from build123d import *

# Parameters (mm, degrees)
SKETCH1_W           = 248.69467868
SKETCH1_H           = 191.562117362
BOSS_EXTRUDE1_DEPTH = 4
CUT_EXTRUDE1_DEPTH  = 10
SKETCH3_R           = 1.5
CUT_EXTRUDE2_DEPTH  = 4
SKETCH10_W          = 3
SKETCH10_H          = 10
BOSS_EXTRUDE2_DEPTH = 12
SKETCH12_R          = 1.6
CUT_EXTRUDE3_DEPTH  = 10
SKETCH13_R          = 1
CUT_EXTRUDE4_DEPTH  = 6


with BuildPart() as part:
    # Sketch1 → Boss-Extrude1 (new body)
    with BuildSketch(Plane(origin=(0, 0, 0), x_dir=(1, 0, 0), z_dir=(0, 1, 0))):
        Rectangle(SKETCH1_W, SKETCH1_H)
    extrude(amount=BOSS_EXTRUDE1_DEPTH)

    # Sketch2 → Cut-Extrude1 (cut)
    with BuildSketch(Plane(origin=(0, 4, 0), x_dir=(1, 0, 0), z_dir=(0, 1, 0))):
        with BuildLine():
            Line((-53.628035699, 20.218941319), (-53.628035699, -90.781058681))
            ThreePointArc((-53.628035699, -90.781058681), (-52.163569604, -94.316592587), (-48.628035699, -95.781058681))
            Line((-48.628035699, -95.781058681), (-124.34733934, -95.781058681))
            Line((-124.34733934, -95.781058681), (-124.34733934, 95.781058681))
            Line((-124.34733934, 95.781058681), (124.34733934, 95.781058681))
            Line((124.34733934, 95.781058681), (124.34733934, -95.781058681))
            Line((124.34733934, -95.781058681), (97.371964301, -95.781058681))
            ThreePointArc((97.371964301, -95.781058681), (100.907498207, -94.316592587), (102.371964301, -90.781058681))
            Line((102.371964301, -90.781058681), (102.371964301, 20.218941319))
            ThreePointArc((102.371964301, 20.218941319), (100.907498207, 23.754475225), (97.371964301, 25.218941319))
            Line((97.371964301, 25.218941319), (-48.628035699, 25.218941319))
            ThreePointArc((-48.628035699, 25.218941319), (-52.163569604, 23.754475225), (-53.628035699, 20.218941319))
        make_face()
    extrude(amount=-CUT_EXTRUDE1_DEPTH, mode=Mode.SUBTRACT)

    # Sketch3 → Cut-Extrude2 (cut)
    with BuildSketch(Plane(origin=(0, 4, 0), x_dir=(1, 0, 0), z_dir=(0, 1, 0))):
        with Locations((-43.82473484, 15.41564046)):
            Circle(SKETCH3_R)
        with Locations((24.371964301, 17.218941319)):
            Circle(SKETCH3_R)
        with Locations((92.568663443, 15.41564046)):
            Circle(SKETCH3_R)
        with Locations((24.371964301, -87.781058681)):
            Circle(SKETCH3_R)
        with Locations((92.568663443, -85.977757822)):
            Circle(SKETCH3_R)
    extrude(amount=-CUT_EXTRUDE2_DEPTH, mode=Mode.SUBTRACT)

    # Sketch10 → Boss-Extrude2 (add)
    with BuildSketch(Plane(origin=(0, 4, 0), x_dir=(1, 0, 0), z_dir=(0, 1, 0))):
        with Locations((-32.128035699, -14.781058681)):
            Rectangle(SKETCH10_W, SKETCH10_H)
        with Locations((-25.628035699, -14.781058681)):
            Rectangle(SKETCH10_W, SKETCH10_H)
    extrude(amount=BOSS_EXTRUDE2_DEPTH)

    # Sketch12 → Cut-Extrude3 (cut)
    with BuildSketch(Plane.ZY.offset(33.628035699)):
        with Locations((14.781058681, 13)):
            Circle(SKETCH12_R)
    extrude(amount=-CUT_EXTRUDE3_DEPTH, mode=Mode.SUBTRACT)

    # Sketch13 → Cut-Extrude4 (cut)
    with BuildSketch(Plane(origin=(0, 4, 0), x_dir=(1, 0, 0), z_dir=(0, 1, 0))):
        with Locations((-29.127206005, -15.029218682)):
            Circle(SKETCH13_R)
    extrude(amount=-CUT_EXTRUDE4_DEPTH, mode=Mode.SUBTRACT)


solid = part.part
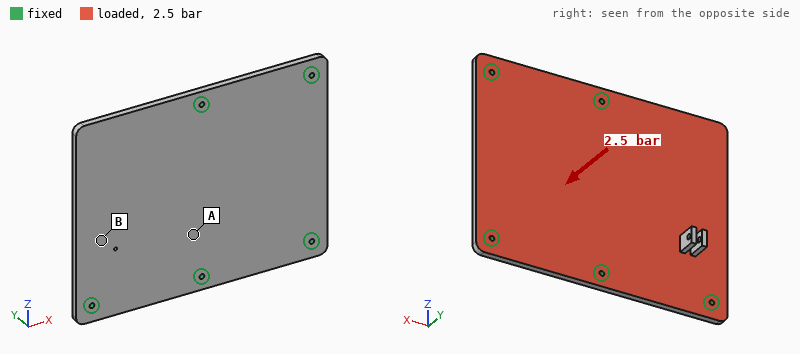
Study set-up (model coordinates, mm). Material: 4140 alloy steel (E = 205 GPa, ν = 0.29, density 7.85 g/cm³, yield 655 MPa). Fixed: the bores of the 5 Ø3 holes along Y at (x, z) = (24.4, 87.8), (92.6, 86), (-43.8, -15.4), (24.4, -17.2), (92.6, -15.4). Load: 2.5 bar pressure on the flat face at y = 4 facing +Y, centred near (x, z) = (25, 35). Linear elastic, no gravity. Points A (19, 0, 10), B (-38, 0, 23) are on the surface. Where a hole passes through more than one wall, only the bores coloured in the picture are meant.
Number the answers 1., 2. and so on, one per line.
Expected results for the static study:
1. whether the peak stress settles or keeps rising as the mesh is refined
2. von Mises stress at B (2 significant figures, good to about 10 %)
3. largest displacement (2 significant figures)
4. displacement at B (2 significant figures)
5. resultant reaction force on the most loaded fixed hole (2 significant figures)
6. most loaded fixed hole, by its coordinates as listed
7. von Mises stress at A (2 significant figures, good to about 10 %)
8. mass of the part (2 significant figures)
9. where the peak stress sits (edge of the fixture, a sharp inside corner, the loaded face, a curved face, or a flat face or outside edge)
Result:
1. keeps rising
2. 75 MPa
3. 0.69 mm
4. 0.25 mm
5. 1.6 kN
6. (24.4, 87.8)
7. 37 MPa
8. 600 g
9. edge of the fixture
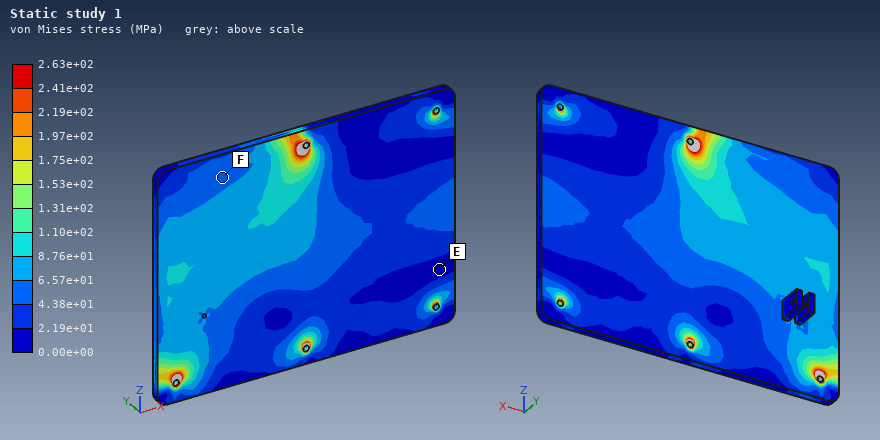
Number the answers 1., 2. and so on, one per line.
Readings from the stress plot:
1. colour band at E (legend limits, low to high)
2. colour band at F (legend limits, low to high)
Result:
1. 0.00e+00 to 2.19e+01 MPa
2. 4.38e+01 to 6.57e+01 MPa
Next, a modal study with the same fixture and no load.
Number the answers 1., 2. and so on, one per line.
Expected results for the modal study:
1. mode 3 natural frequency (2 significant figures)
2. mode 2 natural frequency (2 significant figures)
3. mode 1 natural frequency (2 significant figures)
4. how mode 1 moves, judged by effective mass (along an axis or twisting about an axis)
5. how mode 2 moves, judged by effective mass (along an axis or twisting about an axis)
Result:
1. 1900 Hz
2. 1500 Hz
3. 730 Hz
4. along Y
5. along Y
